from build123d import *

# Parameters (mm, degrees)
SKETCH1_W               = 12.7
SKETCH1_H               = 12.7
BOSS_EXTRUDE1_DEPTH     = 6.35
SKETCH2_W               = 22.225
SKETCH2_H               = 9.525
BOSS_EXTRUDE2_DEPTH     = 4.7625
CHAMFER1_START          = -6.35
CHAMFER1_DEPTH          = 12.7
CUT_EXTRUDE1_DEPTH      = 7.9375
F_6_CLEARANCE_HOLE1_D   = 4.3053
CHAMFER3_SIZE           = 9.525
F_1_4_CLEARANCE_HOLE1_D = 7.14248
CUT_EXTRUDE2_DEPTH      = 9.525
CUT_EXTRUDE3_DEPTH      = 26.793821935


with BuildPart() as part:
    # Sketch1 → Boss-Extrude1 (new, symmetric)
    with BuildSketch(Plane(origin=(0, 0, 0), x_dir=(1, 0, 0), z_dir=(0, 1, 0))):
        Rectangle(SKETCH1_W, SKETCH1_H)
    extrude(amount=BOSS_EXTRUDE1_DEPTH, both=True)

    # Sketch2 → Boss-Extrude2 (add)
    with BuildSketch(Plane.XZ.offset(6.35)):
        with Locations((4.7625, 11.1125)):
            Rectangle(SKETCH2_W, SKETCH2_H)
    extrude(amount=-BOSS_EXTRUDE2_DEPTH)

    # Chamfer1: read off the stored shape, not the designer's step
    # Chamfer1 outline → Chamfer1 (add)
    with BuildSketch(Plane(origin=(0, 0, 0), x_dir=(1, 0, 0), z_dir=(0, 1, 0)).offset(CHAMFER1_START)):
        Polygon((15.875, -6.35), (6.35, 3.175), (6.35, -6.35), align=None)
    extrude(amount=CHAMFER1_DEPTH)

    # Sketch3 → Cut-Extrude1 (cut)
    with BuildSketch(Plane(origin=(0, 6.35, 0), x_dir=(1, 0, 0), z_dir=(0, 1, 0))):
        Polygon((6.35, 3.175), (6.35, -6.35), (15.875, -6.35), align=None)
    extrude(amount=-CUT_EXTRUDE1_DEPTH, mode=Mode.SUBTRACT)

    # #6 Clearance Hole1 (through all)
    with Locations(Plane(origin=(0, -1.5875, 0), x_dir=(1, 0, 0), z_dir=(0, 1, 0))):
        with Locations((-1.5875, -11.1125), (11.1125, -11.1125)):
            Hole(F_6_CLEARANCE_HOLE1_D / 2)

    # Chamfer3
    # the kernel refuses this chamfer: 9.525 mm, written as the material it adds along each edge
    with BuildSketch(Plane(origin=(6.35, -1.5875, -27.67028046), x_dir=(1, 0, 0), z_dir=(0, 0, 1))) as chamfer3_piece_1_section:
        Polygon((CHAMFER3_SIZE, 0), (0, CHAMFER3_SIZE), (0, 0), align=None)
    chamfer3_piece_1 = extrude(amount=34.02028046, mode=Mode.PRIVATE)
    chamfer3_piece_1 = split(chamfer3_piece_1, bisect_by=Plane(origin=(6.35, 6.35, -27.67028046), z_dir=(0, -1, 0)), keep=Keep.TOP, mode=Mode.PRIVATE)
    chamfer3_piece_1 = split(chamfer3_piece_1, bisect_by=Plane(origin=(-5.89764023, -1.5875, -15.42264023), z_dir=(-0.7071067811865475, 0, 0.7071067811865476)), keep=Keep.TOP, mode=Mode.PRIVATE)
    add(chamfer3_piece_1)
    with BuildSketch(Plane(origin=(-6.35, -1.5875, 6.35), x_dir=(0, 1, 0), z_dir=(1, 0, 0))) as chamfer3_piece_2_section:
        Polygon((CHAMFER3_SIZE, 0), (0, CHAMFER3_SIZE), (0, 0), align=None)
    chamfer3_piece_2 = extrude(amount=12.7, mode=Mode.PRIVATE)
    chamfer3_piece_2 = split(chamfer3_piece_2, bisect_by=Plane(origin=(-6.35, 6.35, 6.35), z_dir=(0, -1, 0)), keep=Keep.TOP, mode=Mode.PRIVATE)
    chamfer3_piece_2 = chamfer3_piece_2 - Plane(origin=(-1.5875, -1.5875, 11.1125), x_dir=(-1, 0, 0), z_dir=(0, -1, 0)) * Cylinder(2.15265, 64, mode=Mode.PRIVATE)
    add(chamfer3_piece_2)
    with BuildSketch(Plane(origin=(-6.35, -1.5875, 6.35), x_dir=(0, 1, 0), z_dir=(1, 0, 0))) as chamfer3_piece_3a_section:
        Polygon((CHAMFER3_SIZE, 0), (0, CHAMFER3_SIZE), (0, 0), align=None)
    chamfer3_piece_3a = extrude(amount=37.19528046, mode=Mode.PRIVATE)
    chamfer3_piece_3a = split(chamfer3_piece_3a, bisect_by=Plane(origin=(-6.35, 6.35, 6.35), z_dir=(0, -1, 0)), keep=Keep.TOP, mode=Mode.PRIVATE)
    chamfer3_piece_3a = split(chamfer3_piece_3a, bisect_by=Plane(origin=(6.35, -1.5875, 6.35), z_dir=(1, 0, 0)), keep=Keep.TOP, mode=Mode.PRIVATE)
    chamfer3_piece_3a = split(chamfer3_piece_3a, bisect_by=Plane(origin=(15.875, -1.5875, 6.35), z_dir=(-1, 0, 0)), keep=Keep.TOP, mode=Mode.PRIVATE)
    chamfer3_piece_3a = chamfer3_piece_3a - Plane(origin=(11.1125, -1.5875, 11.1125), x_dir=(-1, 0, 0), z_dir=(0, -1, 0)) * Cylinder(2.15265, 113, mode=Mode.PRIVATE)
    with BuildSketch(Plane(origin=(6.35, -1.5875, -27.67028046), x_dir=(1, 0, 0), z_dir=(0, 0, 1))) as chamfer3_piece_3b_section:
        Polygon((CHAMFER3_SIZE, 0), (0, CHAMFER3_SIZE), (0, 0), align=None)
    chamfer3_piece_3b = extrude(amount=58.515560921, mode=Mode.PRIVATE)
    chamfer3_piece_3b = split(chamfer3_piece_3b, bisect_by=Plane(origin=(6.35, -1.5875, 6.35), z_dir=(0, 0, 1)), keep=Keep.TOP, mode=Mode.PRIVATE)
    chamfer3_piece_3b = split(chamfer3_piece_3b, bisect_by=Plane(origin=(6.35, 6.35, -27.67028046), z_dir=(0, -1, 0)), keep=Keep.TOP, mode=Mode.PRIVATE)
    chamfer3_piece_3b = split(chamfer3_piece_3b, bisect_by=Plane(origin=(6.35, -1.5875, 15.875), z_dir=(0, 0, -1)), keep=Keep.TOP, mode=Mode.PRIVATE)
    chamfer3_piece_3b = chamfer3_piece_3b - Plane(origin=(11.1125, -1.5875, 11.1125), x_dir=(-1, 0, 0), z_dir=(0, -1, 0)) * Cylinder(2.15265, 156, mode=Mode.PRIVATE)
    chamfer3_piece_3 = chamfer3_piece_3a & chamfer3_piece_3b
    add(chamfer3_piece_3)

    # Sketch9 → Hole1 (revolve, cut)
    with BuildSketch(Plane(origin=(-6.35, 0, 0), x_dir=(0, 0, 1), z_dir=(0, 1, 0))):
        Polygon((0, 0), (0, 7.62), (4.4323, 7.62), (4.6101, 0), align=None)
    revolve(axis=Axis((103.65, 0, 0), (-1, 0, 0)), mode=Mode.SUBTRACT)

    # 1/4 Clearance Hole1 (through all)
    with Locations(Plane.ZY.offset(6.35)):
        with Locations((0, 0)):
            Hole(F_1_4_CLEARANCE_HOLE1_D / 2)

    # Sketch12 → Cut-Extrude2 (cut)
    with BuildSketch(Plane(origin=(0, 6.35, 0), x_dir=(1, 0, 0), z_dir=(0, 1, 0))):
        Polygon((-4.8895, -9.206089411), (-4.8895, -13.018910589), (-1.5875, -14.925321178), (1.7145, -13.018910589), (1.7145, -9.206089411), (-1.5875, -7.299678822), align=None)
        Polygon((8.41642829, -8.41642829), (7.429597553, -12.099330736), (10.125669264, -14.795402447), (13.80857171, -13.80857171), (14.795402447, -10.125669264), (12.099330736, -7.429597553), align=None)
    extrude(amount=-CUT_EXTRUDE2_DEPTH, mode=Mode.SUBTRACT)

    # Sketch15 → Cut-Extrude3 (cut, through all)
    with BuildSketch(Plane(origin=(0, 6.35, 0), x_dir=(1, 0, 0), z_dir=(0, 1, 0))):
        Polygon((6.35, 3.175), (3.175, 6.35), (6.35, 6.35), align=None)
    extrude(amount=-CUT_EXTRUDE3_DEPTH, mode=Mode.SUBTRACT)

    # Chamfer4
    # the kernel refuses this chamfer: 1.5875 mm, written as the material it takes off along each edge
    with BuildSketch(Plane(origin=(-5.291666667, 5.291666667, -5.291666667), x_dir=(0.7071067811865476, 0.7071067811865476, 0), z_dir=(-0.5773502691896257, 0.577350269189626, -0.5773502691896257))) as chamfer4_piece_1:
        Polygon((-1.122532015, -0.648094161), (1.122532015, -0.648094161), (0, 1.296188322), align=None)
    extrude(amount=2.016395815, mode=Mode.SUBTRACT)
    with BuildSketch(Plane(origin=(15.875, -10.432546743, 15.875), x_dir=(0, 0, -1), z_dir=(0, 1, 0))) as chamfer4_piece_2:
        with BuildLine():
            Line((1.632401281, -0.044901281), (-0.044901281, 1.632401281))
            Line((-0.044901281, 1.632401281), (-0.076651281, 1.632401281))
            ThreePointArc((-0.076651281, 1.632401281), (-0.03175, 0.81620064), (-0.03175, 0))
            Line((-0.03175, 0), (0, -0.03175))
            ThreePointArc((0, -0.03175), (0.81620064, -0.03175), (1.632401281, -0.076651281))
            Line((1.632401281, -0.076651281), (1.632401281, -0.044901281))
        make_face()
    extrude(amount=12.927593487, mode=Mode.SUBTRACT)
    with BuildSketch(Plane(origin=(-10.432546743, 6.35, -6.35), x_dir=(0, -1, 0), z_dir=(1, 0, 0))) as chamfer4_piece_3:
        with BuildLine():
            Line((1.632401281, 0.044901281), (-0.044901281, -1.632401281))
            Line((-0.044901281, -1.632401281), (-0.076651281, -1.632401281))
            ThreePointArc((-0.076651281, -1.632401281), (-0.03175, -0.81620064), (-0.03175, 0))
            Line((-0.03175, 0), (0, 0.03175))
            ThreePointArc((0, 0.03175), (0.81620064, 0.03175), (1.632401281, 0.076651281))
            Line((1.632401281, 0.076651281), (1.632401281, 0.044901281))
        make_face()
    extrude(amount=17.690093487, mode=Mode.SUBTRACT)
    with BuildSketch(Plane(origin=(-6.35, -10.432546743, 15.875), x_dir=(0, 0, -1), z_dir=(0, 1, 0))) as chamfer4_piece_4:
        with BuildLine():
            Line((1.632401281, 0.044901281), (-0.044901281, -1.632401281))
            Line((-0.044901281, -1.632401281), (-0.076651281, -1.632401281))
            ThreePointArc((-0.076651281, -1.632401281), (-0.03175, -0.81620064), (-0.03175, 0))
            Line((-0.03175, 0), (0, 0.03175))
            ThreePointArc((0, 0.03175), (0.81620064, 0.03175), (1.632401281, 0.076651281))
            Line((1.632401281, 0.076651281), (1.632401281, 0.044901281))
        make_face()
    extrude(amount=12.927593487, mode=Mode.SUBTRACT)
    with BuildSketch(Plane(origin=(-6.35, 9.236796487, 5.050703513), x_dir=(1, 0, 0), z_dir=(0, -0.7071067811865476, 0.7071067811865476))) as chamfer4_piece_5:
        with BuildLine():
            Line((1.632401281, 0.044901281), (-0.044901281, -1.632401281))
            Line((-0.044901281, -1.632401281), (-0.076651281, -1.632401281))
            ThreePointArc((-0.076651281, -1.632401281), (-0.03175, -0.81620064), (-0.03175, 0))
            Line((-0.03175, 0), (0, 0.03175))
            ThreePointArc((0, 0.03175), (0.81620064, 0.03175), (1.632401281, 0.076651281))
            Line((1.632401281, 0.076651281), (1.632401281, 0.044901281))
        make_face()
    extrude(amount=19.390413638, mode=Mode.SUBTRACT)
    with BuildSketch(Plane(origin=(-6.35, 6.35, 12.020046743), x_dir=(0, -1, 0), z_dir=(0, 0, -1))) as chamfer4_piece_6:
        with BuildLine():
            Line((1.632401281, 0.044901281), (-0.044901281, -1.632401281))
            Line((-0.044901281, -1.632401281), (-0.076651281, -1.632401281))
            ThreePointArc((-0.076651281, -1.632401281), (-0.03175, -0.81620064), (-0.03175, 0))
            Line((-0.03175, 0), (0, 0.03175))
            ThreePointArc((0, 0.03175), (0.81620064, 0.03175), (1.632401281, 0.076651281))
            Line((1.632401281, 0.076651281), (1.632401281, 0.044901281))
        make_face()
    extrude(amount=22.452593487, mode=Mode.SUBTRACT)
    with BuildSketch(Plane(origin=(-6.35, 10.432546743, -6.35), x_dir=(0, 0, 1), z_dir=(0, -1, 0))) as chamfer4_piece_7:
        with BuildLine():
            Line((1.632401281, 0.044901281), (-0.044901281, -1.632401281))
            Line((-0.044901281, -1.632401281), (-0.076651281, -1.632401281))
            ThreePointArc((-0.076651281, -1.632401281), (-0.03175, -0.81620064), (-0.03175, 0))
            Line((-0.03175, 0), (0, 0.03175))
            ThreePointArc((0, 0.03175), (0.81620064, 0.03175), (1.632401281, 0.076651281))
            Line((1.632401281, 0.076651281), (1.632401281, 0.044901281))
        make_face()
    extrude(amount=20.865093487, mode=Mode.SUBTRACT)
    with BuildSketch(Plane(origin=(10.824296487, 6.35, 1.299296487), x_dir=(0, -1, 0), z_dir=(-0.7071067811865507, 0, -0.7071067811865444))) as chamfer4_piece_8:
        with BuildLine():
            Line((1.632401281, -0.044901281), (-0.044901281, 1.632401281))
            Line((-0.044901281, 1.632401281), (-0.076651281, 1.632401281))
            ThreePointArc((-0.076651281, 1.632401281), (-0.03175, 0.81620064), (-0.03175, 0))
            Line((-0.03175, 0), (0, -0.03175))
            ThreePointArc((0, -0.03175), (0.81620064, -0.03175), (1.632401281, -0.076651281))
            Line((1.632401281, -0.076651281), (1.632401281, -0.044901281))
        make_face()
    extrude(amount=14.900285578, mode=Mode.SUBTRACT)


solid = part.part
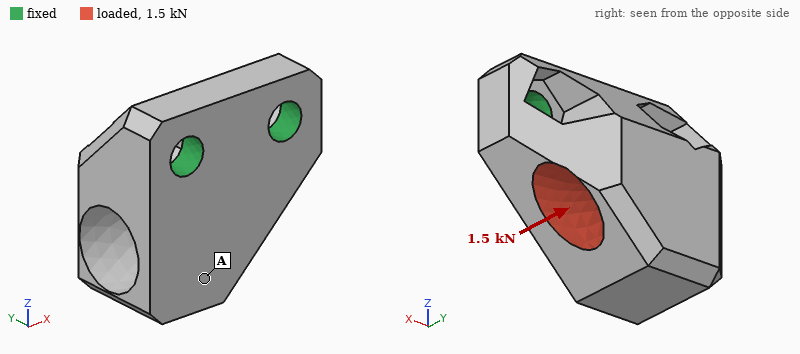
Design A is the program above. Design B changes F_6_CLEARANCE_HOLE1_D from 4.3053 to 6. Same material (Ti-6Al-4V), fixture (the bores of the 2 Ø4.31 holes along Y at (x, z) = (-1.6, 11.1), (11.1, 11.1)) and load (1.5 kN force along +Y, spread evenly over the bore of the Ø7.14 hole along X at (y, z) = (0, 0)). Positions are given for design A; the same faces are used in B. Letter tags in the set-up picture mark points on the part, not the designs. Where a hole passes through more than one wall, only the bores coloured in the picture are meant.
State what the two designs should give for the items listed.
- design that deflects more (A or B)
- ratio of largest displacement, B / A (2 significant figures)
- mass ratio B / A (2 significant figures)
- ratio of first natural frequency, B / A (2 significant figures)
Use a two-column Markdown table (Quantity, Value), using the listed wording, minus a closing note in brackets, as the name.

| Quantity | Value |
|---|---|
| design that deflects more | A |
| ratio of largest displacement, B / A | 0.66 |
| mass ratio B / A | 0.97 |
| ratio of first natural frequency, B / A | 1.2 |
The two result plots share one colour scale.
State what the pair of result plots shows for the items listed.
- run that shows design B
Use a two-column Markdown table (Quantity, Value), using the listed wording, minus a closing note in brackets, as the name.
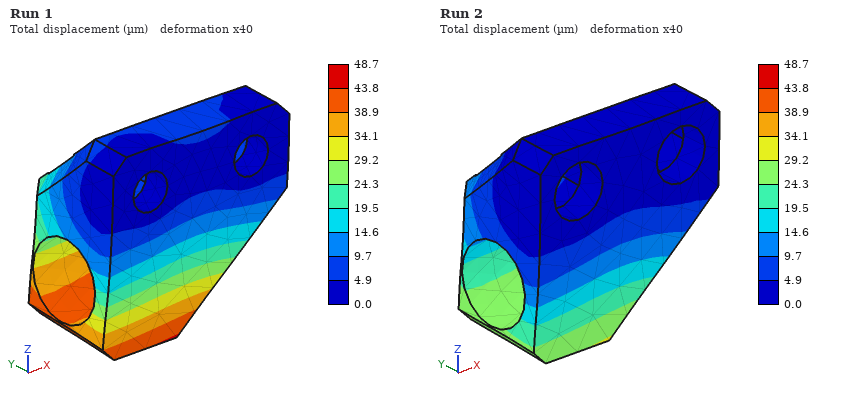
| Quantity | Value |
|---|---|
| run that shows design B | Run 2 |
